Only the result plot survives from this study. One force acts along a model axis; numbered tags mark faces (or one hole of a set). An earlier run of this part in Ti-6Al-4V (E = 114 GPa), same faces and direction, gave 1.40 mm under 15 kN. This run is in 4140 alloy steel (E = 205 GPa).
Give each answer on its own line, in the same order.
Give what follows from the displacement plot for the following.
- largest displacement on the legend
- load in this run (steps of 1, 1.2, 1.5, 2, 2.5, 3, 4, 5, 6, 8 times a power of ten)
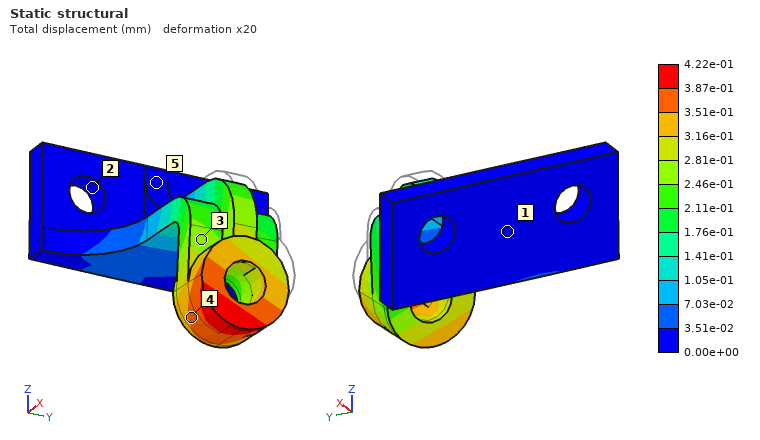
4.22e-01 mm
8 kN
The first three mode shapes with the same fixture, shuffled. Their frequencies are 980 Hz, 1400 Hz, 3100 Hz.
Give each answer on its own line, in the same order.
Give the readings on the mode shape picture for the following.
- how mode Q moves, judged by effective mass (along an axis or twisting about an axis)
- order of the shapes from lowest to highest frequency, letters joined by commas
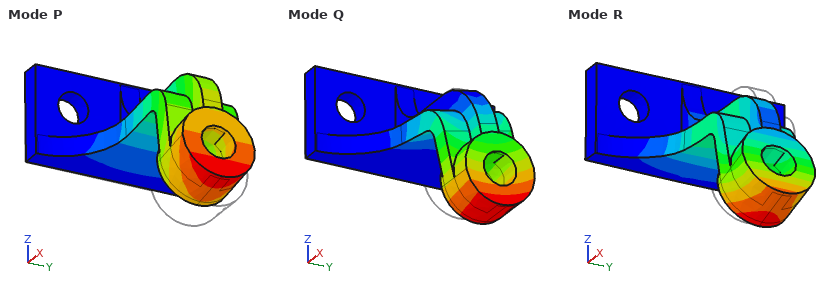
along Y
P, Q, R
